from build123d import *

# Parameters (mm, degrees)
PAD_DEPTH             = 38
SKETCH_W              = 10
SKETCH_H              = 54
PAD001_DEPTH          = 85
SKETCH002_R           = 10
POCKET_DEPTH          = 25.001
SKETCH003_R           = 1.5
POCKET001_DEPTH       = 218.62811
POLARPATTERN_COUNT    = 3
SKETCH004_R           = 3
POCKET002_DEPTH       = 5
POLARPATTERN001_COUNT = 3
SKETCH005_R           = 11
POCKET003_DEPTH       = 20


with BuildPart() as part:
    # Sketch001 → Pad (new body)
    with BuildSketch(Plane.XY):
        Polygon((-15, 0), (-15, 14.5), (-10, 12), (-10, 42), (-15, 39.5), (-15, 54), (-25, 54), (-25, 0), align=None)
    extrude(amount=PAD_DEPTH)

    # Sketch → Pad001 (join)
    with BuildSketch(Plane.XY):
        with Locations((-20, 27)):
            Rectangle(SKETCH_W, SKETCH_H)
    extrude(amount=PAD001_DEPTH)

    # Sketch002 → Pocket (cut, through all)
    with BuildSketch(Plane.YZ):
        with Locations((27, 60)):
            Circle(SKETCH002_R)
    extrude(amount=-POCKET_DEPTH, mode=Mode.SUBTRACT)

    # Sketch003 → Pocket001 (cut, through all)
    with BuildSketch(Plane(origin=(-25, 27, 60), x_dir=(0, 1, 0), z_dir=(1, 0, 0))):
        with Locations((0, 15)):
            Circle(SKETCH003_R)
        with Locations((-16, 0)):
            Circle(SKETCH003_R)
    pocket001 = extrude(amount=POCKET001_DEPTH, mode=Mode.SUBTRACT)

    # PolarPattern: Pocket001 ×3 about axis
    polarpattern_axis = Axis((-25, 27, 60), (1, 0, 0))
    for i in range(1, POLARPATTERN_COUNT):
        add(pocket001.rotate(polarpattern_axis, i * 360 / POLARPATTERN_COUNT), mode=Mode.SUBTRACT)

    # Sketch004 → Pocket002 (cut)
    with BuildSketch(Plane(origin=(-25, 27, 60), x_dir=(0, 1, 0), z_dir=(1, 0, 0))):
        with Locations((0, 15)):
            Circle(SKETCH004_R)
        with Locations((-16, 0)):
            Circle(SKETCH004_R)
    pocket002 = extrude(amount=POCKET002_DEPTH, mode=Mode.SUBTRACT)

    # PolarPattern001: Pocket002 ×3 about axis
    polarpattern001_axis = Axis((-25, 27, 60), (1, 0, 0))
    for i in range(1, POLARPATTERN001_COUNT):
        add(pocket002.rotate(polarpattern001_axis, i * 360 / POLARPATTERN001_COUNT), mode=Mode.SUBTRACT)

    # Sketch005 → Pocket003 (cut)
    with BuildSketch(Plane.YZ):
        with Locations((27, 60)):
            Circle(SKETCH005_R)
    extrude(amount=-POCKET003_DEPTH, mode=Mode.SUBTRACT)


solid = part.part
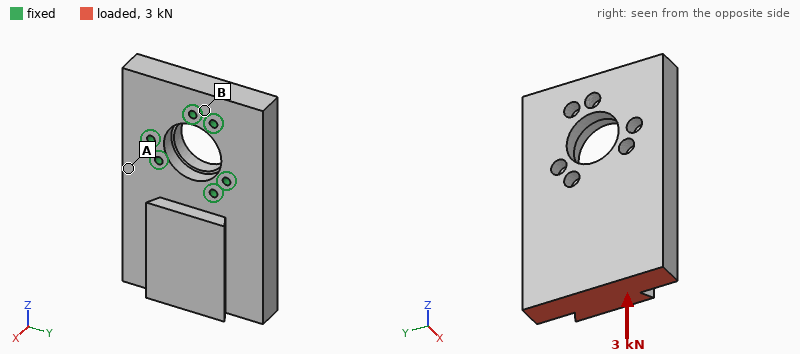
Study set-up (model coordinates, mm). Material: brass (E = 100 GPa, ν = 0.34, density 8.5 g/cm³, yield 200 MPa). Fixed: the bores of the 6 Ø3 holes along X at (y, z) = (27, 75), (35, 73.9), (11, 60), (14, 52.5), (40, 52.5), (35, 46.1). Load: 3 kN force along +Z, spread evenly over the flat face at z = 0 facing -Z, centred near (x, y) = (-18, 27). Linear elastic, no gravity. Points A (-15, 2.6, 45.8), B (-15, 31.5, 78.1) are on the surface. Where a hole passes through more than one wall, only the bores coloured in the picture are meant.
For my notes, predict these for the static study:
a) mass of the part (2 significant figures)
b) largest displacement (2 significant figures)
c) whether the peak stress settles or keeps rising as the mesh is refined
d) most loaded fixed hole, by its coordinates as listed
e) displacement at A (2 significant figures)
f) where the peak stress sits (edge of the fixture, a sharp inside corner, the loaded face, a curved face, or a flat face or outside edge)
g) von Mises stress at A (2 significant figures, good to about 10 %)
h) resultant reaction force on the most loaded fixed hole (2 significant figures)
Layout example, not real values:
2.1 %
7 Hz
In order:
400 g
5.7 µm
keeps rising
(35, 46.1)
1.4 µm
edge of the fixture
6.7 MPa
1.0 kN
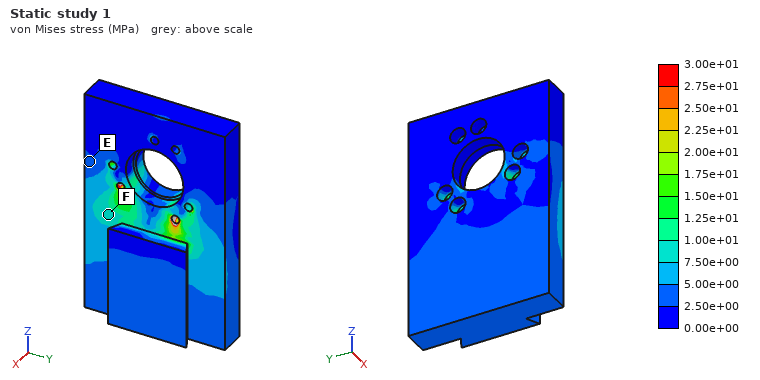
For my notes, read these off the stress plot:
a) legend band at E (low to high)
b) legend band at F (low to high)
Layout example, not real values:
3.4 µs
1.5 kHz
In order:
2.50e+00 to 5.00e+00 MPa
7.50e+00 to 1.00e+01 MPa
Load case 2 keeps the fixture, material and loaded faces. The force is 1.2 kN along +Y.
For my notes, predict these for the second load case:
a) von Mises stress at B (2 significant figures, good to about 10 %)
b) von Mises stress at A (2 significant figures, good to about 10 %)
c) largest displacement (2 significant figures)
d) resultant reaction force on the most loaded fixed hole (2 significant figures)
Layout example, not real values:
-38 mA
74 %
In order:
5.7 MPa
10 MPa
13 µm
1.2 kN
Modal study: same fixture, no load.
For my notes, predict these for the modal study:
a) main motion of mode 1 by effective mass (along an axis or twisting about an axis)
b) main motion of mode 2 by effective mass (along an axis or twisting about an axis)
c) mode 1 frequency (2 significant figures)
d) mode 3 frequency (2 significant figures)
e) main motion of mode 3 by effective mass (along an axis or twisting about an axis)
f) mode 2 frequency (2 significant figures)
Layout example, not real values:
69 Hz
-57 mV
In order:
along X
twisting about Z
1500 Hz
5000 Hz
along Y
4000 Hz
